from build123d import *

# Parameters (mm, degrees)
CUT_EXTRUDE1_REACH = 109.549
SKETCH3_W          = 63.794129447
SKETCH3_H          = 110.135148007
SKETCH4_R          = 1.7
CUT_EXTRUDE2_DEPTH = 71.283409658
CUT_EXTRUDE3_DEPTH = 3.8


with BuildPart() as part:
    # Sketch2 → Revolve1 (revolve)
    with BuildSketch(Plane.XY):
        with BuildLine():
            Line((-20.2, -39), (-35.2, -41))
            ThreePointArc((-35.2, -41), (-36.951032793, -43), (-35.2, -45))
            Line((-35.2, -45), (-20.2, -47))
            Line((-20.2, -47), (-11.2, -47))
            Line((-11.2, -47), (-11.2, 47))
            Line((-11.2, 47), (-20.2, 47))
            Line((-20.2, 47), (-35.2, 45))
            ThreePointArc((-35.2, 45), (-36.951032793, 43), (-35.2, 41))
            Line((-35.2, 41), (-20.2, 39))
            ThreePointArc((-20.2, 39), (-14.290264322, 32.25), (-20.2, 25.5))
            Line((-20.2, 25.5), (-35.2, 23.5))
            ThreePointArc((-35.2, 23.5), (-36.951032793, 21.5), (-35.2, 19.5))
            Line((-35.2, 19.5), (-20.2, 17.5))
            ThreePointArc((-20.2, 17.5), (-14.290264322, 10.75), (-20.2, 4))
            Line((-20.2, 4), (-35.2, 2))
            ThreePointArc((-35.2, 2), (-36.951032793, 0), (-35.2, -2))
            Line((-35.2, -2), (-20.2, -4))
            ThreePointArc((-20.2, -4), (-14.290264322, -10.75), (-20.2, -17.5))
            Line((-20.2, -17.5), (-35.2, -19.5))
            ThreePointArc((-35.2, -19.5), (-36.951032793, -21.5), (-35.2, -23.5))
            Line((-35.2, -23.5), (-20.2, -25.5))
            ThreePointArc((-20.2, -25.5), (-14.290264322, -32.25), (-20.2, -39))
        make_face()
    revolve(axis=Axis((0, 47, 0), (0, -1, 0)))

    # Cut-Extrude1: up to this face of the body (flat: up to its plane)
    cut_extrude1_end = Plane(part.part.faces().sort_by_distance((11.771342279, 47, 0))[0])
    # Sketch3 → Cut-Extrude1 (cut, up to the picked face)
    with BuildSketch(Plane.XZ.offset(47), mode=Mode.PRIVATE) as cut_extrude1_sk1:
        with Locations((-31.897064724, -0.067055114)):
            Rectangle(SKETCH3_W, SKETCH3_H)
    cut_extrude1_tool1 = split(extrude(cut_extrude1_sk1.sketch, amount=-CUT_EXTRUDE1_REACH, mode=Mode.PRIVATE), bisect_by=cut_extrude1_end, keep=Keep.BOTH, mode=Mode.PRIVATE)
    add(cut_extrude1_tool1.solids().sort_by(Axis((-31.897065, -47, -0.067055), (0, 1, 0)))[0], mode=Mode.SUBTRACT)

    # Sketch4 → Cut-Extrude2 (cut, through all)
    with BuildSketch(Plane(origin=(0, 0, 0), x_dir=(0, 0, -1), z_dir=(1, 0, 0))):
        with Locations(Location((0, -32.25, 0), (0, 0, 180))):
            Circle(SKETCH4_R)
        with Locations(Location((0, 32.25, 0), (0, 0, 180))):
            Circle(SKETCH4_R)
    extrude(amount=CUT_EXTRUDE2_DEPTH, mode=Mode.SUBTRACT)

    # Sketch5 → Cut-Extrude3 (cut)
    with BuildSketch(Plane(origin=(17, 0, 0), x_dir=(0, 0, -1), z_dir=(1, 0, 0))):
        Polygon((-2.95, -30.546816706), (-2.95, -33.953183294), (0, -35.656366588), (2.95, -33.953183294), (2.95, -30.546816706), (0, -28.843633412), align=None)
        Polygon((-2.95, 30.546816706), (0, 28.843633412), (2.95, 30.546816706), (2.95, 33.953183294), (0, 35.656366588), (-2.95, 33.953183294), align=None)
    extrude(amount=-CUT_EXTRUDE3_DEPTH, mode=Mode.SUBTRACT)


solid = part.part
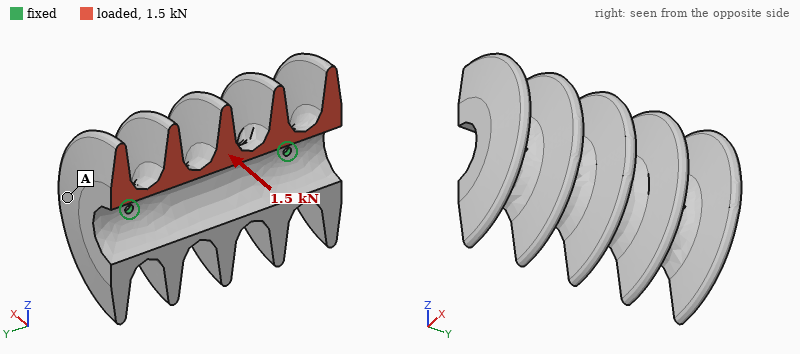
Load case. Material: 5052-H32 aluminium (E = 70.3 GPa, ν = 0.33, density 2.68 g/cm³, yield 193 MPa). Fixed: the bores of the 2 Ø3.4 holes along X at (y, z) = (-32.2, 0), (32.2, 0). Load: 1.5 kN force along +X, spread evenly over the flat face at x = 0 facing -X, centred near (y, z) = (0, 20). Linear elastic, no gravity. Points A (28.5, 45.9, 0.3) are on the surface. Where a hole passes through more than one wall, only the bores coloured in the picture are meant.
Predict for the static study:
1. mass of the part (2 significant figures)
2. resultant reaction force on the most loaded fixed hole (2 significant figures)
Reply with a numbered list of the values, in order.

1. 190 g
2. 750 N
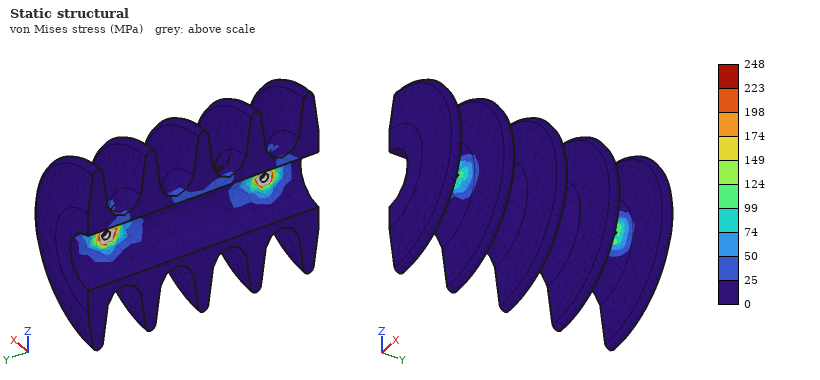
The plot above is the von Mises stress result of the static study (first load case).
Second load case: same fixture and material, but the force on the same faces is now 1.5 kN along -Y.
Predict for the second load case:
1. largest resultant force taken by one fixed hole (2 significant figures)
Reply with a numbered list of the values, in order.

1. 920 N
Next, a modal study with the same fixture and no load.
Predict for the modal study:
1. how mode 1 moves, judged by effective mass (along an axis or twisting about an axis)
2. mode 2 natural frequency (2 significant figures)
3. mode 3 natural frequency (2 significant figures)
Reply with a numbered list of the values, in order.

1. twisting about Y
2. 1900 Hz
3. 3100 Hz
